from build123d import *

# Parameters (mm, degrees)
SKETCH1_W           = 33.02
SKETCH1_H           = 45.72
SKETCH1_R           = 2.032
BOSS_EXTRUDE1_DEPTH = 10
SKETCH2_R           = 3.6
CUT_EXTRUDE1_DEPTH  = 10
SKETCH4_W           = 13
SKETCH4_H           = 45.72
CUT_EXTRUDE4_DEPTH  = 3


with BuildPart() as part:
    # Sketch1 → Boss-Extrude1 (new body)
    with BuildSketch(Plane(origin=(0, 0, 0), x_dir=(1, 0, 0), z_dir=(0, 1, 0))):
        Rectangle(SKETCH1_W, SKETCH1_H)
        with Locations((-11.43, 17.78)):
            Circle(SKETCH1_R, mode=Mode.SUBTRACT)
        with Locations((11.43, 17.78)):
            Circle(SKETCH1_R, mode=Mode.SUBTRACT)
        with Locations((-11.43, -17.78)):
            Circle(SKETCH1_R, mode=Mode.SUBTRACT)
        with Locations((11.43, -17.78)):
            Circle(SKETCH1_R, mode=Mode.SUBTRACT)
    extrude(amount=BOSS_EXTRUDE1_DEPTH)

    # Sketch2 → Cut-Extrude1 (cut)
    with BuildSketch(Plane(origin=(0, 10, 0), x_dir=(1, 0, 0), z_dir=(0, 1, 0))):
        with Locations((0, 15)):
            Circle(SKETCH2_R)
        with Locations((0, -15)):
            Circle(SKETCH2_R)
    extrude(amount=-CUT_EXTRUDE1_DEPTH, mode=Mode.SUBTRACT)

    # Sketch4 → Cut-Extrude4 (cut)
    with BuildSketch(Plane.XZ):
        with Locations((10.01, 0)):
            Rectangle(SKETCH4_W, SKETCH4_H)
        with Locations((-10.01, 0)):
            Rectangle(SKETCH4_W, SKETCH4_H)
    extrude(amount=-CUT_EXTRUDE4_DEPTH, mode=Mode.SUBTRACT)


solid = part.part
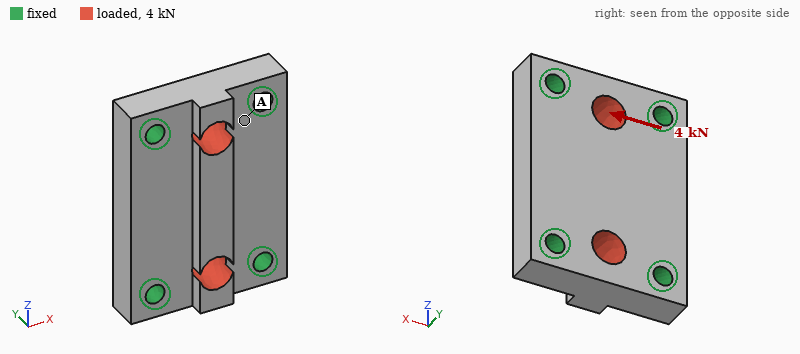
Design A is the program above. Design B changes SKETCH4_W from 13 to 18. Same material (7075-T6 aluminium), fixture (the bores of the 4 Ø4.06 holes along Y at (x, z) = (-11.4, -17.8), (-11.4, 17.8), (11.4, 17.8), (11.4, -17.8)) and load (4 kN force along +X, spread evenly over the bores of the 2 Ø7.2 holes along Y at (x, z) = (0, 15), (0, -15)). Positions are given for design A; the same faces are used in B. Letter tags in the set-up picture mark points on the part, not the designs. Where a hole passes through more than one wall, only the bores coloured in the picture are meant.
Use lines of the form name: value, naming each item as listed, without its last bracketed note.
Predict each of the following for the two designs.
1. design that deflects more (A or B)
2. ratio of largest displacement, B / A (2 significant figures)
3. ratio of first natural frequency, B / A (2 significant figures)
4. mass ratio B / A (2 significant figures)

design that deflects more: A
ratio of largest displacement, B / A: 0.25
ratio of first natural frequency, B / A: 1.00
mass ratio B / A: 0.95
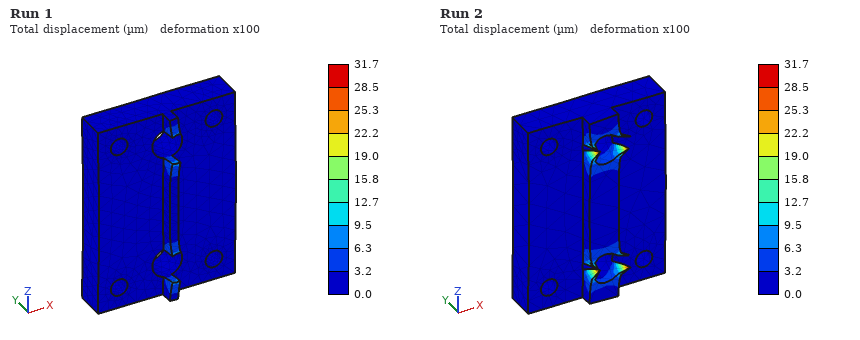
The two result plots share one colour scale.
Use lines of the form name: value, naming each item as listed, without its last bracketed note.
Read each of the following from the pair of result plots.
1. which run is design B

which run is design B: Run 1
